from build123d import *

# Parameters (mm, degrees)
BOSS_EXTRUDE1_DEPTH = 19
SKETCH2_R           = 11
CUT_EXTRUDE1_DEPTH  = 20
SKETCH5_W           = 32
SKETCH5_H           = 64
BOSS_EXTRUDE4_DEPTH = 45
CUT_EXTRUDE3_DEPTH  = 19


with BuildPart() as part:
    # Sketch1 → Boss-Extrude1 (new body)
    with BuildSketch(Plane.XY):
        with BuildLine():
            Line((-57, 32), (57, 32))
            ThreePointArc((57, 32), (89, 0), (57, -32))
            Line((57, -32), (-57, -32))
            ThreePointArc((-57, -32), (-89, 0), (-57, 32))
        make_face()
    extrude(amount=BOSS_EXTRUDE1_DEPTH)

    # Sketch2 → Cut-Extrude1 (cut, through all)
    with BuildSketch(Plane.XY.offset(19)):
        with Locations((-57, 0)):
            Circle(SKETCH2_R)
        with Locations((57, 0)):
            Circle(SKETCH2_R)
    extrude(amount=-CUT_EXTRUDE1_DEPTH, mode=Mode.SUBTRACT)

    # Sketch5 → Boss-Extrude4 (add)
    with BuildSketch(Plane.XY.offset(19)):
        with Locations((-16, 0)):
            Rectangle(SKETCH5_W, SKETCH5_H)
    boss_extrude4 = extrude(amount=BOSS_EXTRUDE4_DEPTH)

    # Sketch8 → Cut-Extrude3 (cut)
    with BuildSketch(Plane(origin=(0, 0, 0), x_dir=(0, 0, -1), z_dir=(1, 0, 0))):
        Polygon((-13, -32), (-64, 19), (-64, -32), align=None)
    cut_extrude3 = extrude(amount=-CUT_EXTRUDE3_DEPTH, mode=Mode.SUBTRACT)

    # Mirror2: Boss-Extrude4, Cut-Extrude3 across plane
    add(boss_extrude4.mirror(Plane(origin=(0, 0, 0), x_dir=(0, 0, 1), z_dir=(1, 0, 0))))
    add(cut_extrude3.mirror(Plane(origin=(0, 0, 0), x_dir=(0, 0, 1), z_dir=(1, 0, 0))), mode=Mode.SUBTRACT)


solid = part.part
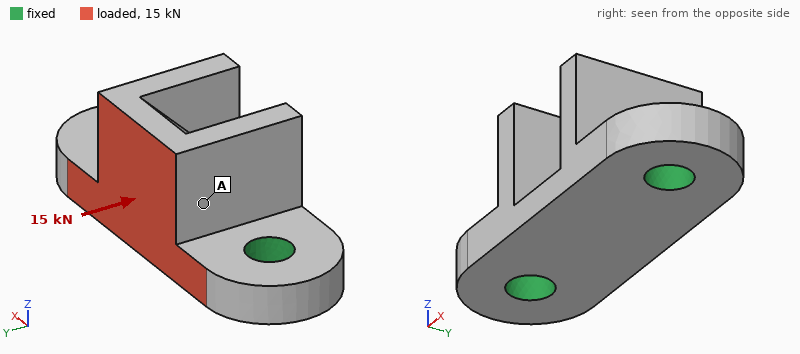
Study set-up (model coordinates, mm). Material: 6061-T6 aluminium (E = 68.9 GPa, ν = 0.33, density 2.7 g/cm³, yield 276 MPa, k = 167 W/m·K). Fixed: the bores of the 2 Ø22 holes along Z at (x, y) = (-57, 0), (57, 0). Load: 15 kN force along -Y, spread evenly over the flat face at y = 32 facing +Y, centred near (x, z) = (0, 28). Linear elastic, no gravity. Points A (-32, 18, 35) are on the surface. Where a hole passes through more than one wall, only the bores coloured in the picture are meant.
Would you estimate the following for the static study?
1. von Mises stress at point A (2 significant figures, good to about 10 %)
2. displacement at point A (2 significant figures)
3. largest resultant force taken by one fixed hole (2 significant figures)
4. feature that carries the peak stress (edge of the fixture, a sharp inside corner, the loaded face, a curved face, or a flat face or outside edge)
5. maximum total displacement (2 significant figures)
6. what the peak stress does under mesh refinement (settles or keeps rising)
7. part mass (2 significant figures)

7.0 MPa
35 µm
7.5 kN
edge of the fixture
67 µm
keeps rising
860 g
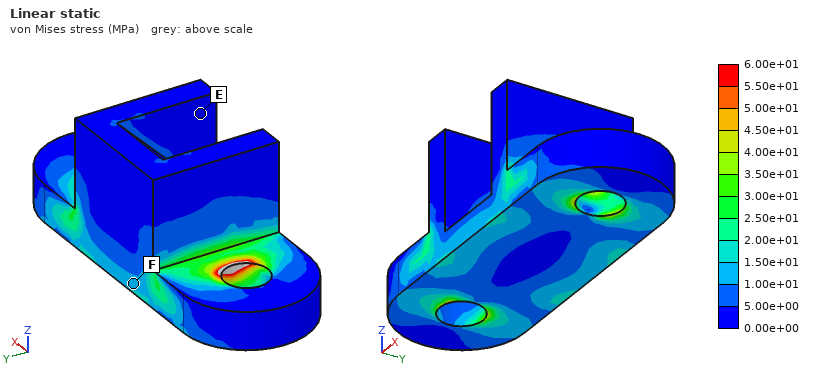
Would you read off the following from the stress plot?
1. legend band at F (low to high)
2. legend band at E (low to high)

1.00e+01 to 1.50e+01 MPa
0.00e+00 to 5.00e+00 MPa
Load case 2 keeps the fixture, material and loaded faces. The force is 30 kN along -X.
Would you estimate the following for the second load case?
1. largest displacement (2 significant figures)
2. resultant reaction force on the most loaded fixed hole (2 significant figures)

46 µm
18 kN
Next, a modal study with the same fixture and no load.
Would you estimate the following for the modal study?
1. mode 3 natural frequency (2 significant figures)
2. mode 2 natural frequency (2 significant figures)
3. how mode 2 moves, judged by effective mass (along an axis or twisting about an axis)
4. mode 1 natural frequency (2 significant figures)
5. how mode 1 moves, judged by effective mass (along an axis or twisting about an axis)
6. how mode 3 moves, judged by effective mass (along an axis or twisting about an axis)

7000 Hz
6300 Hz
along Z
3500 Hz
along Y
along X
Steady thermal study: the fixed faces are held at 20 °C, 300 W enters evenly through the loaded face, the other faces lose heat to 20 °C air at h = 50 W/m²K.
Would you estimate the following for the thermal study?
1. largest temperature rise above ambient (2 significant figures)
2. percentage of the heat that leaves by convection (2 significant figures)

34 K
7.9 %
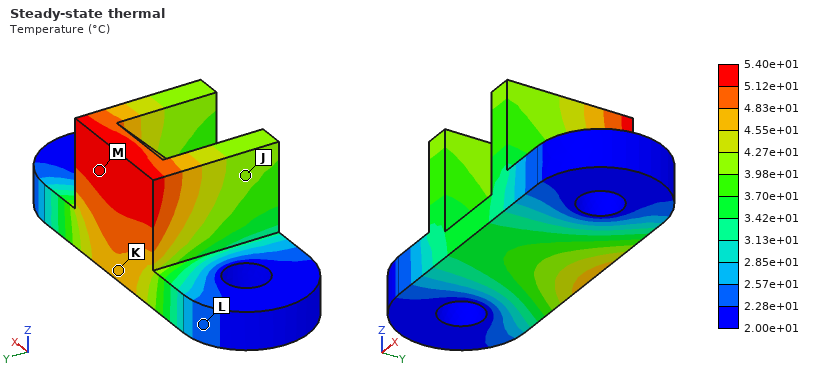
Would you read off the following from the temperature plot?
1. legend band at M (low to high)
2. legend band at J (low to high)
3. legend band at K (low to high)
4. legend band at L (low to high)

5.12e+01 to 5.40e+01 °C
3.98e+01 to 4.27e+01 °C
4.55e+01 to 4.83e+01 °C
2.28e+01 to 2.57e+01 °C
